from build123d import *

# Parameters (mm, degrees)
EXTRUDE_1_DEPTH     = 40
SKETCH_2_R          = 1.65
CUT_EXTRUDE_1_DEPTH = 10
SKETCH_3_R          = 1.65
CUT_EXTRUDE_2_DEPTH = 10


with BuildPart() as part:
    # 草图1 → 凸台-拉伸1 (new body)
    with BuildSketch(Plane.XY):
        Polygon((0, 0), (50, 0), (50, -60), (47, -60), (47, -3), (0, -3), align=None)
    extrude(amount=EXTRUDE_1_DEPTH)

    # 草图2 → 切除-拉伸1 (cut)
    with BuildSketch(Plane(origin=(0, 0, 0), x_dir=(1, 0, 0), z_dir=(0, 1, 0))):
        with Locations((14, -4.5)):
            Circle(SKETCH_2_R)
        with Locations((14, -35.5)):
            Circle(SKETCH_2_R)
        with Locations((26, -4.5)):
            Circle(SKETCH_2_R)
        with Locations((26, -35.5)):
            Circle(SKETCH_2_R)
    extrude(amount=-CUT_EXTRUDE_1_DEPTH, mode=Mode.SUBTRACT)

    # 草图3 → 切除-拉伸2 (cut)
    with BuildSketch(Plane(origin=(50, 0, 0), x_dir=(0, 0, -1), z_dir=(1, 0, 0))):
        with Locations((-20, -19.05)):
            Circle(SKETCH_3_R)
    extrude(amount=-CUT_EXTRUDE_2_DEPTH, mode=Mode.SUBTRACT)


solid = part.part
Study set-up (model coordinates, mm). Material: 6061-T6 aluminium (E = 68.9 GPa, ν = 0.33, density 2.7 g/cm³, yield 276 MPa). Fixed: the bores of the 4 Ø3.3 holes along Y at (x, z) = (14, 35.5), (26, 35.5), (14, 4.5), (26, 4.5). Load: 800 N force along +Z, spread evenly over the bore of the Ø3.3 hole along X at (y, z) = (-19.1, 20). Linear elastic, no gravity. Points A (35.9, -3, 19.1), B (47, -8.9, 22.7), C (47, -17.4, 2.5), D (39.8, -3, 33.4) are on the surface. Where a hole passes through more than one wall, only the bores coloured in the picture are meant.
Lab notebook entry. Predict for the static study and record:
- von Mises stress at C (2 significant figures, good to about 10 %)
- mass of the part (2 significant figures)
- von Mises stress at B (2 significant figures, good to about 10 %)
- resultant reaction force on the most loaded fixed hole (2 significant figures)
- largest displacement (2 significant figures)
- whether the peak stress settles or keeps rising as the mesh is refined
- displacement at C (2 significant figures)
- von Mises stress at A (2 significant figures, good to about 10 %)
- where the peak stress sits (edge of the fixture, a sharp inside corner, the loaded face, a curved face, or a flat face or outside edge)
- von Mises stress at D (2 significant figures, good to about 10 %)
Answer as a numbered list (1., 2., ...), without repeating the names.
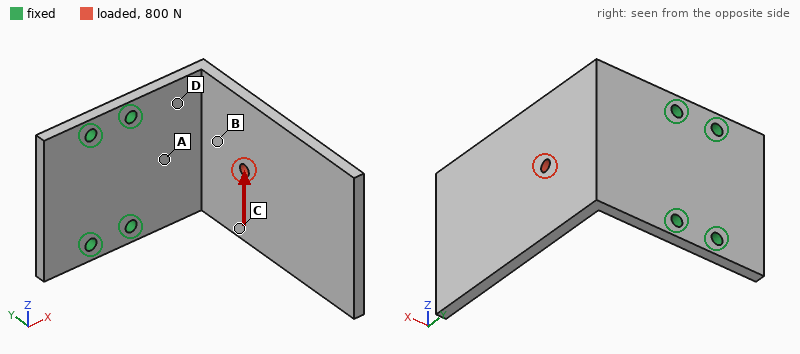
1. 31 MPa
2. 34 g
3. 55 MPa
4. 790 N
5. 0.92 mm
6. keeps rising
7. 0.36 mm
8. 110 MPa
9. edge of the fixture
10. 120 MPa
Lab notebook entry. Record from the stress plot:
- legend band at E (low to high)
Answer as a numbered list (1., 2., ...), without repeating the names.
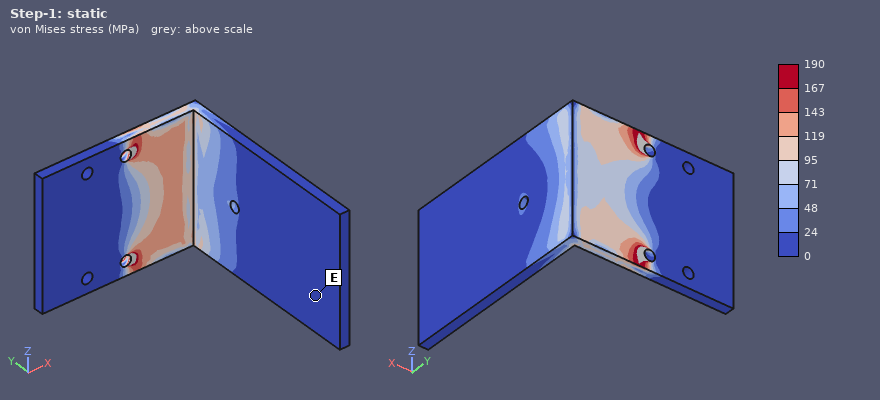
1. 0 to 24 MPa
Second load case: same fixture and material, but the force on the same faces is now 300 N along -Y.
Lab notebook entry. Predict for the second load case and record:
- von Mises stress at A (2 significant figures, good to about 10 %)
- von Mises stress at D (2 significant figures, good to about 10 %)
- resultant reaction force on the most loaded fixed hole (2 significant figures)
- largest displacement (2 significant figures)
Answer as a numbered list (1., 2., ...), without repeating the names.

1. 53 MPa
2. 42 MPa
3. 240 N
4. 0.76 mm
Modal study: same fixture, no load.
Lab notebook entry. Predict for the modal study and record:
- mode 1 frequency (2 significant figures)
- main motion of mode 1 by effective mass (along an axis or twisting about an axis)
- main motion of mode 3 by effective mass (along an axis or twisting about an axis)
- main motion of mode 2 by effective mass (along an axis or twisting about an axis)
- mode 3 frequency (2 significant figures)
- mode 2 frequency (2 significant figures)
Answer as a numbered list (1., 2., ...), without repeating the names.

1. 450 Hz
2. along X
3. along Y
4. along Z
5. 1800 Hz
6. 990 Hz
